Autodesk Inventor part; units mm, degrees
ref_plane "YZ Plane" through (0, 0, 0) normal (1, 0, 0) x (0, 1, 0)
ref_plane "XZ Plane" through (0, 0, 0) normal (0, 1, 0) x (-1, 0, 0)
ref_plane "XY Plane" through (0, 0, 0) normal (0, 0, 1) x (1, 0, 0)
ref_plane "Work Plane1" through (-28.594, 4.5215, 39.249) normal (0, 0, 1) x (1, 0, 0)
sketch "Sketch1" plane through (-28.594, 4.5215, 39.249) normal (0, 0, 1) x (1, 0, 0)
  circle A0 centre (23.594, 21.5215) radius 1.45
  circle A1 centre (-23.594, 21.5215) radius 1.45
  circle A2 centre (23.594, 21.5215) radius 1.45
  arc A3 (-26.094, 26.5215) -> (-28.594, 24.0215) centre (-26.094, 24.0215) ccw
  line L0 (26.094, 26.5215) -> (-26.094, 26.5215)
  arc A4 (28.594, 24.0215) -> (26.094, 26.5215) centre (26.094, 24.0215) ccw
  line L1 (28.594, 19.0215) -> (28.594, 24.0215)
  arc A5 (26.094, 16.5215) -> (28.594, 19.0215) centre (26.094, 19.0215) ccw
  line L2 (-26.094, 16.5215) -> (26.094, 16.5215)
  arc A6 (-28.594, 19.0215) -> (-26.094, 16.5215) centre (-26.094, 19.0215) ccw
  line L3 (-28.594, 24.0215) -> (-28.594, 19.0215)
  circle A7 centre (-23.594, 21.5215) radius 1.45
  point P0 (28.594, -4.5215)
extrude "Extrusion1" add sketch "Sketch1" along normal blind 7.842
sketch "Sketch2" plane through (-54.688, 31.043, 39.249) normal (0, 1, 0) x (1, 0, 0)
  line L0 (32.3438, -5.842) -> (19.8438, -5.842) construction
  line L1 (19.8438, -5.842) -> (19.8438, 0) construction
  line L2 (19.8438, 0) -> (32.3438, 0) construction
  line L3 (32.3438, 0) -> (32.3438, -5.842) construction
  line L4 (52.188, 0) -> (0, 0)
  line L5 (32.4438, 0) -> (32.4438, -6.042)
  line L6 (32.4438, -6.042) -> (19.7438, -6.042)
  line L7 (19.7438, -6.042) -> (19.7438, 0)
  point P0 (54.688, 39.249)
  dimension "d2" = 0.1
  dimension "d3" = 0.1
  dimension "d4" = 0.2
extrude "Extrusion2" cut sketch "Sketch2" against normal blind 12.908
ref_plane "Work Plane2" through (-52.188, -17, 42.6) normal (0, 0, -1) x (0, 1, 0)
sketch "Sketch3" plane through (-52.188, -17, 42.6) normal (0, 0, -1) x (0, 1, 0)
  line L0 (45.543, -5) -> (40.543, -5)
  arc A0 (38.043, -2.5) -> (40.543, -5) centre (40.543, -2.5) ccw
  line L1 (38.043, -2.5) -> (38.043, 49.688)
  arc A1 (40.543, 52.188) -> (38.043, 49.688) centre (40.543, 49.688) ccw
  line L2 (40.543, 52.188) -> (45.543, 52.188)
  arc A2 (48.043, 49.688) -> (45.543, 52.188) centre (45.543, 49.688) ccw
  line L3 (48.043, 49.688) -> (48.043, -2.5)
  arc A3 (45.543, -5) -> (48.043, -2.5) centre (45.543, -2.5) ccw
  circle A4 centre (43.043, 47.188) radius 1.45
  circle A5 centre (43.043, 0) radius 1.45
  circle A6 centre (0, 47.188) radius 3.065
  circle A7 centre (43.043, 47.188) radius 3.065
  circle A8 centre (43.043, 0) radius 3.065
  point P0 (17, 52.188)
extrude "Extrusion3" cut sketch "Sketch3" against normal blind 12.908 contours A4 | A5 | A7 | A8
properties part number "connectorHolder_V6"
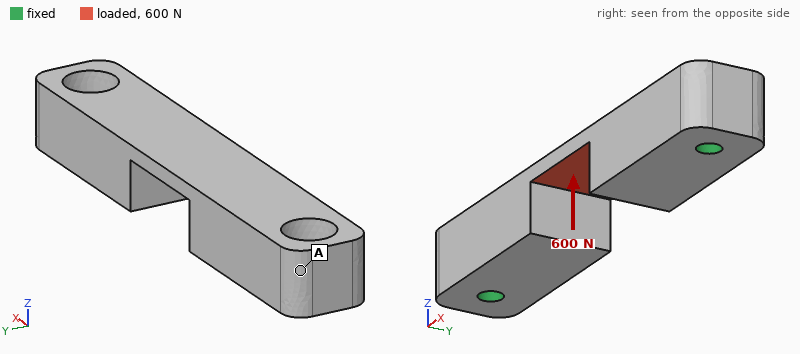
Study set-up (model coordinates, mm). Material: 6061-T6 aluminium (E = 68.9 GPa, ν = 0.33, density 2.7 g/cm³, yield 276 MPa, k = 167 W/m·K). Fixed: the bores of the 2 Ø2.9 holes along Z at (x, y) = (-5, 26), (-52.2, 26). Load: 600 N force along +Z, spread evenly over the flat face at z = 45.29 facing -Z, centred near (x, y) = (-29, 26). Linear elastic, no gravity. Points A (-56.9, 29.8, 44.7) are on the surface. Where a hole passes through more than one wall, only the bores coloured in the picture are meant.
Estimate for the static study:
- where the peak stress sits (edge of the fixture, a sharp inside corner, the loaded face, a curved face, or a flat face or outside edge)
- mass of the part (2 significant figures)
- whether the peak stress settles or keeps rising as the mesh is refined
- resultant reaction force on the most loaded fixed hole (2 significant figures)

edge of the fixture
9.1 g
keeps rising
770 N
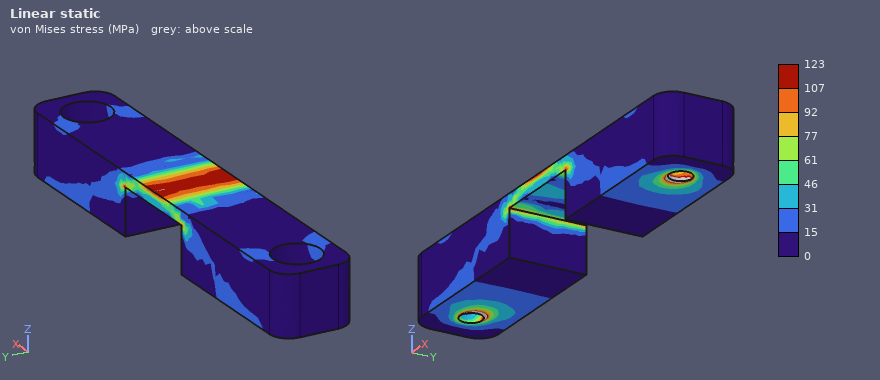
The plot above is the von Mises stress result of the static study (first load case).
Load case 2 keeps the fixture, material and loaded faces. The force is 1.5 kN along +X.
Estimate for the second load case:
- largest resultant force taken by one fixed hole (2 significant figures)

750 N
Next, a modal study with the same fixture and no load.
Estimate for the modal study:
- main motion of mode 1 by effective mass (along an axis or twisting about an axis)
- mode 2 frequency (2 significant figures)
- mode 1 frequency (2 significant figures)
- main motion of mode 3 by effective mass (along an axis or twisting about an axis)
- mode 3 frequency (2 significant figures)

along Y
13 kHz
12 kHz
along Z
14 kHz
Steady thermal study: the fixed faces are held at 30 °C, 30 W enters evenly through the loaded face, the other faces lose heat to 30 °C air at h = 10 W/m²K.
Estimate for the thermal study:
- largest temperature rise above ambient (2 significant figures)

46 K
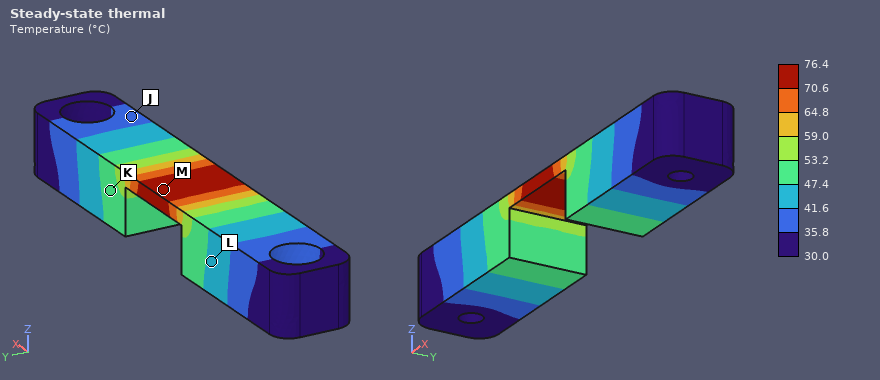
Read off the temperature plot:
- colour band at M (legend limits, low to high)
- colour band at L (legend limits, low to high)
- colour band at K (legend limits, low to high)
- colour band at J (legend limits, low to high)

70.6 to 76.4 °C
41.6 to 47.4 °C
47.4 to 53.2 °C
35.8 to 41.6 °C
